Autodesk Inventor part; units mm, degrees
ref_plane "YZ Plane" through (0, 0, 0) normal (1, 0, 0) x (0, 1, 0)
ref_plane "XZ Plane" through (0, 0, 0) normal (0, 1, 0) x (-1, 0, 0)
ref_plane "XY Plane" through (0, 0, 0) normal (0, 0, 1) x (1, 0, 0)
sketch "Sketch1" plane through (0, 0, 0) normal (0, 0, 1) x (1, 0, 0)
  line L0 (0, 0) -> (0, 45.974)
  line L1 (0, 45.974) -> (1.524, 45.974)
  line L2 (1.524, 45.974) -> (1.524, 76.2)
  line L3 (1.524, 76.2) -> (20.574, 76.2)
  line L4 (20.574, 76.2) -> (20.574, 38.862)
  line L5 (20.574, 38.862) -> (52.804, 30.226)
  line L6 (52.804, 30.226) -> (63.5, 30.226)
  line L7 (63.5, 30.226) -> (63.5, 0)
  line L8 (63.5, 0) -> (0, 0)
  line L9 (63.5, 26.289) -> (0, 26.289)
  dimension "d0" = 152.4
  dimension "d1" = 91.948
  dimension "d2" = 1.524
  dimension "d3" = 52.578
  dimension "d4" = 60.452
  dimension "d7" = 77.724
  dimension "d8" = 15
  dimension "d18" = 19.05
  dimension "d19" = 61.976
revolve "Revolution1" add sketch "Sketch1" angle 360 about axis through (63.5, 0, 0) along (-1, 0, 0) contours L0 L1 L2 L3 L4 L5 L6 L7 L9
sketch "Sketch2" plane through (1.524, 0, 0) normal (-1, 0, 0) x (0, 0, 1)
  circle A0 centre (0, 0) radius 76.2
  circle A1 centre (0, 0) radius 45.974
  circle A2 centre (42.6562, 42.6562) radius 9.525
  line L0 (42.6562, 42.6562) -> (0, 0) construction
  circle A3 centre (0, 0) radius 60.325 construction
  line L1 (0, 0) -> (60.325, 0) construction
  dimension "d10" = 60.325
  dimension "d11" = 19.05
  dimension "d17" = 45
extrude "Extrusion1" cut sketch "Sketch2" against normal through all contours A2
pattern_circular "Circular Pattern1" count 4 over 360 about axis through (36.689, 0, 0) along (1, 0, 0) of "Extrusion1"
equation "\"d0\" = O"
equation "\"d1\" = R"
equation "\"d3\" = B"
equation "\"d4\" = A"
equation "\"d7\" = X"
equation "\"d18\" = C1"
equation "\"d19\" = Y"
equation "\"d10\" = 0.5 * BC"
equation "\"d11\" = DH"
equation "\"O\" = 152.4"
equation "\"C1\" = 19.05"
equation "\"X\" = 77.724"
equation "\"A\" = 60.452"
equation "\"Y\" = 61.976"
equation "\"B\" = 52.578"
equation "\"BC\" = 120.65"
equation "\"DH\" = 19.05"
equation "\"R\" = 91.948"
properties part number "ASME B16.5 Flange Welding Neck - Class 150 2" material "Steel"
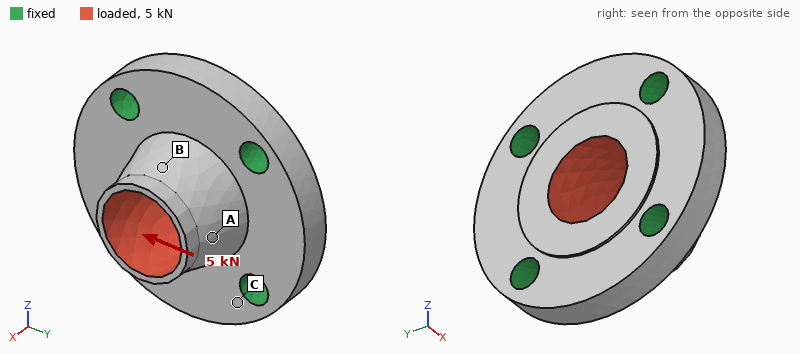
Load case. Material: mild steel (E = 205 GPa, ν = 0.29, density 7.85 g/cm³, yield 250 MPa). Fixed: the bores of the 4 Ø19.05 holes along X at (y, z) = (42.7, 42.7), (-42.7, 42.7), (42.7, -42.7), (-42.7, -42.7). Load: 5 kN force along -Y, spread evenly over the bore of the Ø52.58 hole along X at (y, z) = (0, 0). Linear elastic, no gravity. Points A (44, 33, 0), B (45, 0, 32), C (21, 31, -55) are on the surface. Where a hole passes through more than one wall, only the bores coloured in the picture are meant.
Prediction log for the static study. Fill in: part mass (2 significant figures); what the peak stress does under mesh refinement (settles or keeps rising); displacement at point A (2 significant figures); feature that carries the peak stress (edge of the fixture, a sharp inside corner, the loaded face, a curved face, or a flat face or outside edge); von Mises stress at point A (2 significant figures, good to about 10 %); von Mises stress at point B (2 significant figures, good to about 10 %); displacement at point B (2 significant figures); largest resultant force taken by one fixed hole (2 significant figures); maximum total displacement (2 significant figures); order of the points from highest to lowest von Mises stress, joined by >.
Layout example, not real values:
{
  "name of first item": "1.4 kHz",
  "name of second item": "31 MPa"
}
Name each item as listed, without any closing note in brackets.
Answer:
{
  "part mass": "2.7 kg",
  "what the peak stress does under mesh refinement": "keeps rising",
  "displacement at point A": "1.7 µm",
  "feature that carries the peak stress": "edge of the fixture",
  "von Mises stress at point A": "2.4 MPa",
  "von Mises stress at point B": "3.4 MPa",
  "displacement at point B": "1.2 µm",
  "largest resultant force taken by one fixed hole": "1.4 kN",
  "maximum total displacement": "2.6 µm",
  "order of the points from highest to lowest von Mises stress, joined by >": "B > A > C"
}
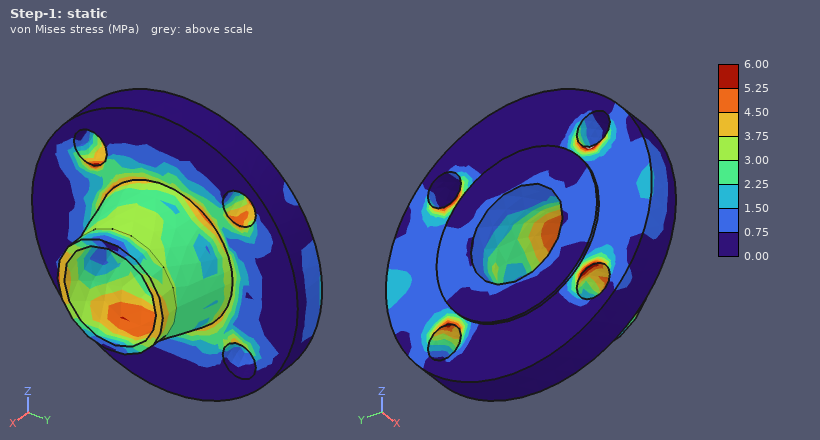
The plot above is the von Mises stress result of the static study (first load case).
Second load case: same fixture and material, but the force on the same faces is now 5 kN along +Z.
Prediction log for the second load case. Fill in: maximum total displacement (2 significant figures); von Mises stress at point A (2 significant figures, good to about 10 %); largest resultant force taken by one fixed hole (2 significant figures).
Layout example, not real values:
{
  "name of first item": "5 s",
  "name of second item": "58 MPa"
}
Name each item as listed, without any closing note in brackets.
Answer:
{
  "maximum total displacement": "2.6 µm",
  "von Mises stress at point A": "3.4 MPa",
  "largest resultant force taken by one fixed hole": "1.4 kN"
}
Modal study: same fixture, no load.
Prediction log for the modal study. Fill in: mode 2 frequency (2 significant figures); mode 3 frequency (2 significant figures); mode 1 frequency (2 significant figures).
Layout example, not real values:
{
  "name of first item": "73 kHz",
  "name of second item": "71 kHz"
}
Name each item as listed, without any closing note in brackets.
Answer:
{
  "mode 2 frequency": "10 kHz",
  "mode 3 frequency": "10 kHz",
  "mode 1 frequency": "9400 Hz"
}
